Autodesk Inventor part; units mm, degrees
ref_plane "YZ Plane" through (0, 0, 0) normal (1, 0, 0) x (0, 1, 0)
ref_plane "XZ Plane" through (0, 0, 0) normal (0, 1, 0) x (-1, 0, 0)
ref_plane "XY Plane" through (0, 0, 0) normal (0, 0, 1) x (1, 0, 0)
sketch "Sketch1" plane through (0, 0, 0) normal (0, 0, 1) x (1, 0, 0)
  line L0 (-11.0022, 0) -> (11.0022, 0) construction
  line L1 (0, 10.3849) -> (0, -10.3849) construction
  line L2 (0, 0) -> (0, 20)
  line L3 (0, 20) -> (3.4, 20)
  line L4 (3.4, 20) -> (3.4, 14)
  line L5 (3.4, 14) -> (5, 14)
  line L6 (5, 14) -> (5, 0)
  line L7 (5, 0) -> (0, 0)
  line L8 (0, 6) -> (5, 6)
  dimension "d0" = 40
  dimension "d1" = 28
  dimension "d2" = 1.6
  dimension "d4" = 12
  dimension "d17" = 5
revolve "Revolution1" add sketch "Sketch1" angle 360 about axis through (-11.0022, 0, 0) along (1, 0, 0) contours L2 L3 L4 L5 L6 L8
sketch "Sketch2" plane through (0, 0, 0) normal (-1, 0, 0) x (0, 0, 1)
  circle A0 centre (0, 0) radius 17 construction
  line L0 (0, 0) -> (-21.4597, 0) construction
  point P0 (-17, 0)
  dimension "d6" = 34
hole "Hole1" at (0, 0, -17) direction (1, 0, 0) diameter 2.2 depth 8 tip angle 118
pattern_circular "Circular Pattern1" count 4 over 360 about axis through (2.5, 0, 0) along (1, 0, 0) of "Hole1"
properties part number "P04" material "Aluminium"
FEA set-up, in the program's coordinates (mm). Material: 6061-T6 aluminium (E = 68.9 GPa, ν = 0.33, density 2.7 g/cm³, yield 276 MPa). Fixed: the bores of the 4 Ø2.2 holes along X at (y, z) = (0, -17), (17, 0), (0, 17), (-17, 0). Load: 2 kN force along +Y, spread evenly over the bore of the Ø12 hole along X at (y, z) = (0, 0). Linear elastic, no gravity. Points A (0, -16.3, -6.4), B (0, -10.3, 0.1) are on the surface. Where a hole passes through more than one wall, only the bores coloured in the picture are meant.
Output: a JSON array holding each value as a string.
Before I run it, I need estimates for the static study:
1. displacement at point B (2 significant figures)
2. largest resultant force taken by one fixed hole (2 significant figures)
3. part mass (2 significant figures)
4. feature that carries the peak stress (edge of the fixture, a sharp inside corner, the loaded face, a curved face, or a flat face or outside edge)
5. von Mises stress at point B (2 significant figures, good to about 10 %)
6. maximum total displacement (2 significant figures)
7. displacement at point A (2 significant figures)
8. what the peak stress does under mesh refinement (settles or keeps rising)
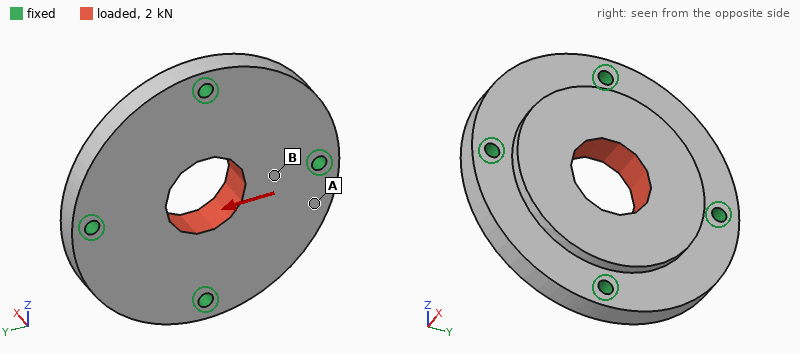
["1.9 µm", "620 N", "13 g", "edge of the fixture", "18 MPa", "3.6 µm", "1.8 µm", "keeps rising"]
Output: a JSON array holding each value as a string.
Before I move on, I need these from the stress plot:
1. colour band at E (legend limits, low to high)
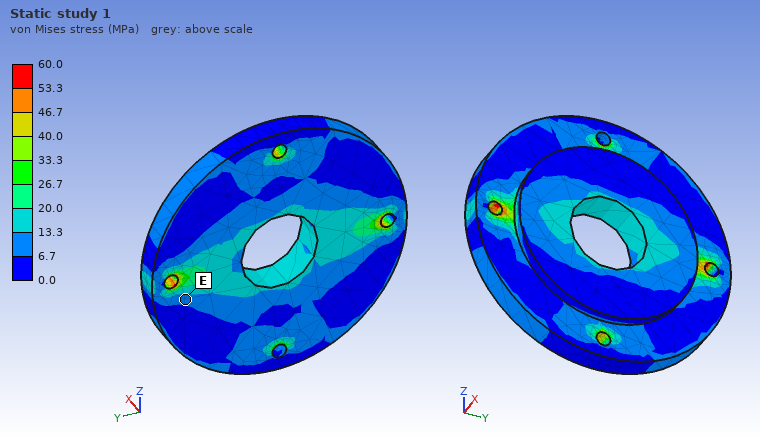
["6.7 to 13.3 MPa"]
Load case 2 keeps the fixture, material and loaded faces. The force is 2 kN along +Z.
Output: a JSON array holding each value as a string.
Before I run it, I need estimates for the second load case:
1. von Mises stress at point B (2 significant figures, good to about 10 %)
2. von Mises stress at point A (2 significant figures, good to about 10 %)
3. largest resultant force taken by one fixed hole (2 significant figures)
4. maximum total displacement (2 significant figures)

["5.4 MPa", "7.2 MPa", "620 N", "3.6 µm"]
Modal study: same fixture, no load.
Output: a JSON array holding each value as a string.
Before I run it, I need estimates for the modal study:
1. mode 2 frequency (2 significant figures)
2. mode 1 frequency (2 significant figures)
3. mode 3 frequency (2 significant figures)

["23 kHz", "22 kHz", "25 kHz"]
